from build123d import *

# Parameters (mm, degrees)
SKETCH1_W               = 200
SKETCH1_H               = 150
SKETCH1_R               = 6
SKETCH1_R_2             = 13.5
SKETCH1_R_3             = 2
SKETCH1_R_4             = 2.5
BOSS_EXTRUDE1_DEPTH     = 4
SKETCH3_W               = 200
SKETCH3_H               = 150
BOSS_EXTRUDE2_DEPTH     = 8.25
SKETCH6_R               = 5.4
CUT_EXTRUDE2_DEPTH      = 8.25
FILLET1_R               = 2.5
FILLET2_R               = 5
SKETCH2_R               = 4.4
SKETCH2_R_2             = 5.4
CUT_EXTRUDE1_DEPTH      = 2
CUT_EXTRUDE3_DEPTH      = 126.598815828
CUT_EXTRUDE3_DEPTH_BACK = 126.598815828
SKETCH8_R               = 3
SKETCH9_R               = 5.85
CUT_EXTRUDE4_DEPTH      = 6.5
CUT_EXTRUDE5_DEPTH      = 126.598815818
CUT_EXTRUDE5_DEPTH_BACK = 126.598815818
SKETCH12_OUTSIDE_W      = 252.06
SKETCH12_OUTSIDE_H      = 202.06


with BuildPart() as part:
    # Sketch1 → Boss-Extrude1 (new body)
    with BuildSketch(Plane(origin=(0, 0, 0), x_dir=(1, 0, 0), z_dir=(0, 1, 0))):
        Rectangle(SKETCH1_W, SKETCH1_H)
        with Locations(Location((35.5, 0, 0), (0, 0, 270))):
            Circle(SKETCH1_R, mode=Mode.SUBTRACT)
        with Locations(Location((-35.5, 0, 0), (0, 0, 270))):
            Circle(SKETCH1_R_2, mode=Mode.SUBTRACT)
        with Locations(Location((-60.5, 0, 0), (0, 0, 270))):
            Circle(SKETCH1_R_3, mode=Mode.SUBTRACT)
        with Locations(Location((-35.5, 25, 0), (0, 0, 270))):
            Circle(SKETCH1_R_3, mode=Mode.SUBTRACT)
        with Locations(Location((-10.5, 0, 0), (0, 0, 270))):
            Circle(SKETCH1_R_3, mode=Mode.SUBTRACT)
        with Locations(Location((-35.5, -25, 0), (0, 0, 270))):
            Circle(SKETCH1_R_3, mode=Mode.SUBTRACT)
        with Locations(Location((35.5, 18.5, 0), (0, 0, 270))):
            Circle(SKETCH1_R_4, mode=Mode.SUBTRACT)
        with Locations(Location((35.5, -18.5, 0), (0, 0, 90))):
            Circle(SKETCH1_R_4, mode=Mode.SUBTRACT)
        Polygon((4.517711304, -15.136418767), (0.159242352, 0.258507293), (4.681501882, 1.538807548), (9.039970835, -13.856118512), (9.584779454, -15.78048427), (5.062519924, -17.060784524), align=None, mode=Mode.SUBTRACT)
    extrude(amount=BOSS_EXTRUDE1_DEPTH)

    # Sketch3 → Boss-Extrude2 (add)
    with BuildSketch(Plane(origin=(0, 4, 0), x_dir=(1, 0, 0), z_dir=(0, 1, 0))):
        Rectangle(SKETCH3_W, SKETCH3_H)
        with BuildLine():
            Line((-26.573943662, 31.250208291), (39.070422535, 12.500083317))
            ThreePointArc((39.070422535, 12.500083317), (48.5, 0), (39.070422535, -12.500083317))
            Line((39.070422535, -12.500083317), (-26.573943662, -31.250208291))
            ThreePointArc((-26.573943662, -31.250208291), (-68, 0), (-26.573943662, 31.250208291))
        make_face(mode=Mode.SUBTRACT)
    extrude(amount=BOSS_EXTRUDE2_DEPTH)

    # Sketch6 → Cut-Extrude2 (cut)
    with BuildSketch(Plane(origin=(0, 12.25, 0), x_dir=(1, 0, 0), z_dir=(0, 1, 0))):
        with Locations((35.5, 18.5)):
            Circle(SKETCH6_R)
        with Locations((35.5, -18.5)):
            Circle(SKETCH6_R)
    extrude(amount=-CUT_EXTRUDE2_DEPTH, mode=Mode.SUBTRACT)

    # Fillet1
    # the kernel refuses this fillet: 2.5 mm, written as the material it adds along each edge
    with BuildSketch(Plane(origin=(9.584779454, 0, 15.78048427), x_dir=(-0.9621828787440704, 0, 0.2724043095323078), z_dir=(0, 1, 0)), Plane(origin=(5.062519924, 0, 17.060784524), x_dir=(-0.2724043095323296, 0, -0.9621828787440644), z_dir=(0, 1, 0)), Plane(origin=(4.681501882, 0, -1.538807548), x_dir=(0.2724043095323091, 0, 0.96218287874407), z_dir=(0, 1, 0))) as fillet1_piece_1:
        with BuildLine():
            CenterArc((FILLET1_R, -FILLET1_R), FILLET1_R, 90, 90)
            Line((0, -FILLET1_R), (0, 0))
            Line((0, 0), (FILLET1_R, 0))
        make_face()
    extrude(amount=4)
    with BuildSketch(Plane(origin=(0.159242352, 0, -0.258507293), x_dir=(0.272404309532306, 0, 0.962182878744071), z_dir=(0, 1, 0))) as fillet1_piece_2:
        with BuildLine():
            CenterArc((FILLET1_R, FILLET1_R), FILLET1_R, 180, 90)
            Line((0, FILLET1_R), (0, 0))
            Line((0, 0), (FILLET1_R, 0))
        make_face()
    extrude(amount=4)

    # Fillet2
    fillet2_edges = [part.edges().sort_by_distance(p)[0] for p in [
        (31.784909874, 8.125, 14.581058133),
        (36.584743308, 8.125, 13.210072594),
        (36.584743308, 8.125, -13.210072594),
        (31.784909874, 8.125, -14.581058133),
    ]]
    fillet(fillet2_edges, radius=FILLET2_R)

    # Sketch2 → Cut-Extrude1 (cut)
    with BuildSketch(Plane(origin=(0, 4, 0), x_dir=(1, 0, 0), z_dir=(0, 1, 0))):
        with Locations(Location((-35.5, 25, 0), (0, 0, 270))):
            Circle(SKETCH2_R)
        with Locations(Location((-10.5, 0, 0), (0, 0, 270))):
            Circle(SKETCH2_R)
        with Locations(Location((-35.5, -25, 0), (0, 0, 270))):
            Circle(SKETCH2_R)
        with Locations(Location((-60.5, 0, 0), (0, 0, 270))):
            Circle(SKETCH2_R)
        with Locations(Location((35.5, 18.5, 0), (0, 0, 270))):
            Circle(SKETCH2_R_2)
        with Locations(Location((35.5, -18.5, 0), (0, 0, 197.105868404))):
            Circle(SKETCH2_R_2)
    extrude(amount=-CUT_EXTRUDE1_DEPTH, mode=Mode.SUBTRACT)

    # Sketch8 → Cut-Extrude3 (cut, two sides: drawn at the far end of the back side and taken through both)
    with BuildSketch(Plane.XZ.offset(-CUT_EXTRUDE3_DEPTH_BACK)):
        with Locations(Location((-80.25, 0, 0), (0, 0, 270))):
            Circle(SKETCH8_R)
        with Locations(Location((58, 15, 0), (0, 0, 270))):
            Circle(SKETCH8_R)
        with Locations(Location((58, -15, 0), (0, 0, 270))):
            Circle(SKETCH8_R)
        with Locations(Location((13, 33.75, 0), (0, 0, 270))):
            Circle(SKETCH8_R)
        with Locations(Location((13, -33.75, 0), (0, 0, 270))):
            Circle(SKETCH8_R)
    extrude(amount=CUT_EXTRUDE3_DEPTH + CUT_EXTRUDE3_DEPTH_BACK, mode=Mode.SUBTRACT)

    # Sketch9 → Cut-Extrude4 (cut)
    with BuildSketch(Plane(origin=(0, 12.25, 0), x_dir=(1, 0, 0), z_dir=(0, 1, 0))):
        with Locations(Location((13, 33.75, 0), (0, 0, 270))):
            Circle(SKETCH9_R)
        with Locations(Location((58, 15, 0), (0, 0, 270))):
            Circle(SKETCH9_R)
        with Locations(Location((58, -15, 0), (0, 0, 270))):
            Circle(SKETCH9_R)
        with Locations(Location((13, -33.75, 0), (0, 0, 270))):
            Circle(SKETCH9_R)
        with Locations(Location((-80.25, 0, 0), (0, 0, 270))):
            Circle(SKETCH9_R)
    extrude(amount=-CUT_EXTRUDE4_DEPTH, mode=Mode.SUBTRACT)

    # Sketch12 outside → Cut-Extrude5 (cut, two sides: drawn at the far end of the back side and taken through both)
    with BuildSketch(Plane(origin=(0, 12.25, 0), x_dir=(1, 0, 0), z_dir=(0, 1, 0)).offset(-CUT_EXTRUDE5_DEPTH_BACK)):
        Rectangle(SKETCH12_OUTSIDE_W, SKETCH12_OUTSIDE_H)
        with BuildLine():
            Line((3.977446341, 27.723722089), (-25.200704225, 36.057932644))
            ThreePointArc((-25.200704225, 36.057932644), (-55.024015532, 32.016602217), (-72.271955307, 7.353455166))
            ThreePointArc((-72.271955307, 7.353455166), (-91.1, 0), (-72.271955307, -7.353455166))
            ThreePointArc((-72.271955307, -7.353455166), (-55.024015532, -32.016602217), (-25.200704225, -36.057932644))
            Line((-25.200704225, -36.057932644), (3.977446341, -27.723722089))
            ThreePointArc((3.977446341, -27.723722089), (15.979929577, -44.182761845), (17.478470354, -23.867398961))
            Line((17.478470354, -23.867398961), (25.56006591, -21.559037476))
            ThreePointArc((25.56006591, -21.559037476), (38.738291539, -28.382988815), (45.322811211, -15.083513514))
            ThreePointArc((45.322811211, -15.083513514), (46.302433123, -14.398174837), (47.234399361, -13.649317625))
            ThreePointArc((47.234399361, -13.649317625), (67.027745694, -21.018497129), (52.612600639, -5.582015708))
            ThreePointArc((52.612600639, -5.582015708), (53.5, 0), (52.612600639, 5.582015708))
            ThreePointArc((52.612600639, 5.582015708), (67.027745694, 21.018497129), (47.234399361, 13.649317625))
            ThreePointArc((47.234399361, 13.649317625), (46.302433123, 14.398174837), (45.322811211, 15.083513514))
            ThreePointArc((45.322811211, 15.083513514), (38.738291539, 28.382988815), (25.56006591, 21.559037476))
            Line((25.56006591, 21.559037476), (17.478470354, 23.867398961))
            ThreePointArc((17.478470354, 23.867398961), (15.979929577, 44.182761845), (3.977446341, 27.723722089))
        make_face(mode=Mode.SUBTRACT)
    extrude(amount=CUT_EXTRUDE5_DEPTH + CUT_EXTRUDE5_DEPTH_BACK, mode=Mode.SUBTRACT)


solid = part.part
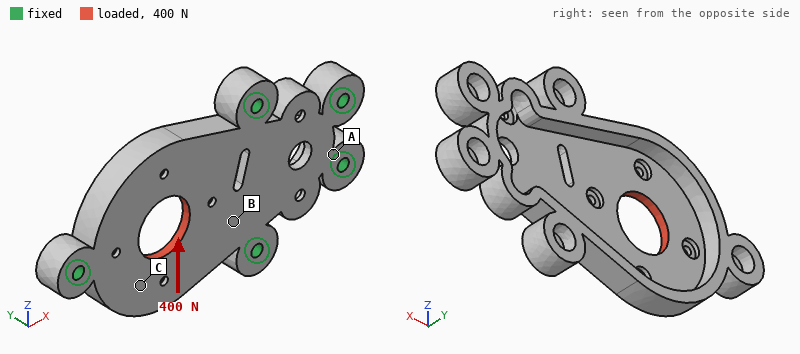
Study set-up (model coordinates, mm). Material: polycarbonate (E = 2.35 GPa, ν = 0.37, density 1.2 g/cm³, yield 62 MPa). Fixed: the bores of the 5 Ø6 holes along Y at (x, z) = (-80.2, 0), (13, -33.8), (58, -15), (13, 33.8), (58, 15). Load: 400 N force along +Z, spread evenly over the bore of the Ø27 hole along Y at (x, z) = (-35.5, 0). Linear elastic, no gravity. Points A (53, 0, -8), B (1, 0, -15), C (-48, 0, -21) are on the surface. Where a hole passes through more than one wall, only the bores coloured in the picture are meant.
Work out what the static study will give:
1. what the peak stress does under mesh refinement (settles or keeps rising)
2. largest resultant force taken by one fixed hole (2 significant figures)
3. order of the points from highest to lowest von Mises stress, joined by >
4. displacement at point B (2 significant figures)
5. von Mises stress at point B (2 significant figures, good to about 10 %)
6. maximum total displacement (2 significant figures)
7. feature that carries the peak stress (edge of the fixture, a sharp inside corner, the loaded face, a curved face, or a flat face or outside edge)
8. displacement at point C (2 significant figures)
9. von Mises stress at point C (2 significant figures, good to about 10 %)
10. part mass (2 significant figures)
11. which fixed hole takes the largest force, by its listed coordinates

keeps rising
180 N
B > C > A
19 µm
1.8 MPa
76 µm
edge of the fixture
62 µm
0.99 MPa
66 g
(-80.2, 0)
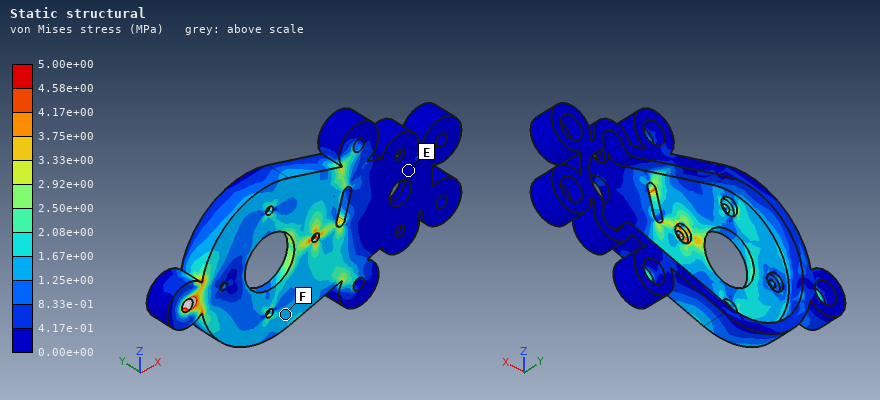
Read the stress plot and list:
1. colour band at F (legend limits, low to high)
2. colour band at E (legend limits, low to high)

1.25e+00 to 1.67e+00 MPa
0.00e+00 to 4.17e-01 MPa
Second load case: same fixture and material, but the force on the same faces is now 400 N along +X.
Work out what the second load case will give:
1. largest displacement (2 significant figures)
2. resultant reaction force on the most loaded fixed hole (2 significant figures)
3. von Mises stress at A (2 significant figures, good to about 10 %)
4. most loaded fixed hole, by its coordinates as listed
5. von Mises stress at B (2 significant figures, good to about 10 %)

32 µm
170 N
0.44 MPa
(-80.2, 0)
0.87 MPa
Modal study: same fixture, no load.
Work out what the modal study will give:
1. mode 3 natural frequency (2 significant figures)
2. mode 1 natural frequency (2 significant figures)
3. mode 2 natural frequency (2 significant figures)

1500 Hz
970 Hz
1000 Hz
